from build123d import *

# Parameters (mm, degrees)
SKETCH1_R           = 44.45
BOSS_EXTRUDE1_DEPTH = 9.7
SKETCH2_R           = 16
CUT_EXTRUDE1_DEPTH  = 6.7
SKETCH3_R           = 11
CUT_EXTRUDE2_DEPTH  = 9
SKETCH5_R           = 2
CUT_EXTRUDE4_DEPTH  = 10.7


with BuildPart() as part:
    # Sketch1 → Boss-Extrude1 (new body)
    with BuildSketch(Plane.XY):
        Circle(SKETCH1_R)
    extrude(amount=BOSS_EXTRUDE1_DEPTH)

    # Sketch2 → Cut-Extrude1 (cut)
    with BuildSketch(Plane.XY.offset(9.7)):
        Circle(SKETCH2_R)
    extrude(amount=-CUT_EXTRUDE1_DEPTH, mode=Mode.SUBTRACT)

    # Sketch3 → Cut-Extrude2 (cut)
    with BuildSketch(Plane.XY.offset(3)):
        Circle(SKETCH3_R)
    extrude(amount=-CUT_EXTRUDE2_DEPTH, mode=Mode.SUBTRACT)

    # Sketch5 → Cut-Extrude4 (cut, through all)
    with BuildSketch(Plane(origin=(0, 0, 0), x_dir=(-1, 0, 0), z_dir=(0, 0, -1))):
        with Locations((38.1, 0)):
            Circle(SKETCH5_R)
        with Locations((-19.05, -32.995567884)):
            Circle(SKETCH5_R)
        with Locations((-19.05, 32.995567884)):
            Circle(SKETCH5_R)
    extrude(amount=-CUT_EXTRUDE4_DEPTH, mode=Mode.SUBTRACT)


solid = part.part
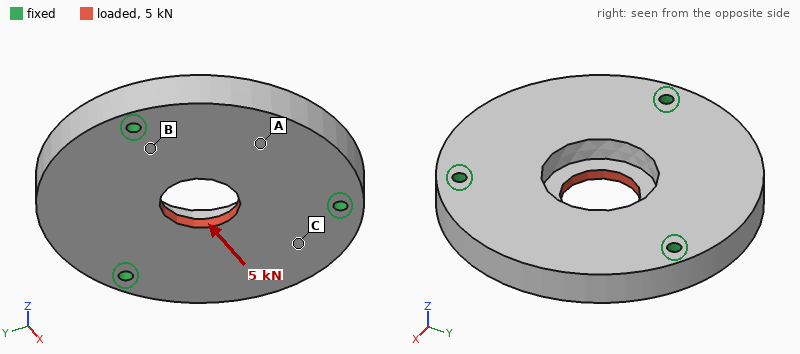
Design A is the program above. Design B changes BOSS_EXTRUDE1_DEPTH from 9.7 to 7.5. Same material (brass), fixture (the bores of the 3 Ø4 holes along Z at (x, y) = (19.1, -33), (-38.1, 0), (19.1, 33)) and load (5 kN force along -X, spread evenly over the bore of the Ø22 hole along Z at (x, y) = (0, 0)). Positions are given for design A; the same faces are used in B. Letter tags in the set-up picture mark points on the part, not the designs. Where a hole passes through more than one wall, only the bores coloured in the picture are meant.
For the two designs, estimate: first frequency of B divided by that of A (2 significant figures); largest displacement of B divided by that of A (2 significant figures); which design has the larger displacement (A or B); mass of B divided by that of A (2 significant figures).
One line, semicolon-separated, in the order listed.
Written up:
0.82; 1.1; B; 0.78
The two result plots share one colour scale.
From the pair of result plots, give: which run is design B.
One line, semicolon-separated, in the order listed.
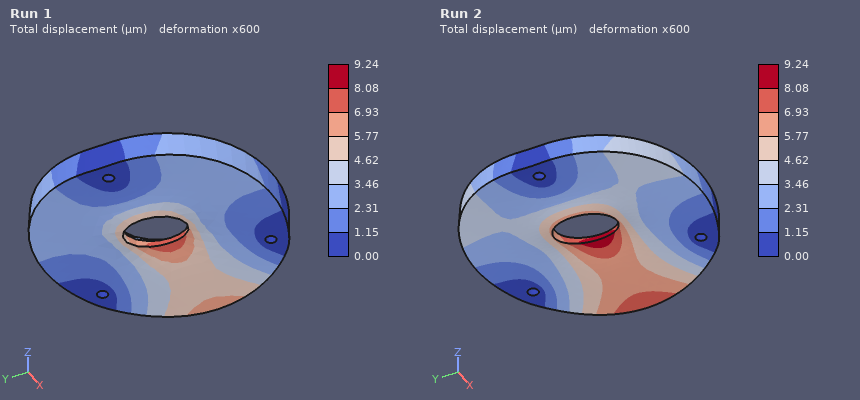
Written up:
Run 2
